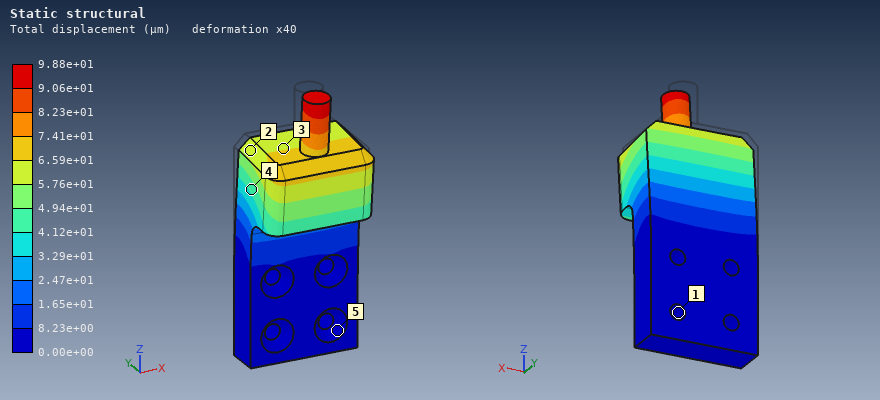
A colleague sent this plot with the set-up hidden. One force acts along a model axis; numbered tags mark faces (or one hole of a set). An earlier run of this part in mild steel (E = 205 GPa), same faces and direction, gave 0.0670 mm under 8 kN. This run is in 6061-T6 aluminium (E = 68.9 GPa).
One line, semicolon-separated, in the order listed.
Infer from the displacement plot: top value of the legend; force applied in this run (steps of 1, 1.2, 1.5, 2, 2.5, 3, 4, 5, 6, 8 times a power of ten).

9.88e+01 µm; 4 kN
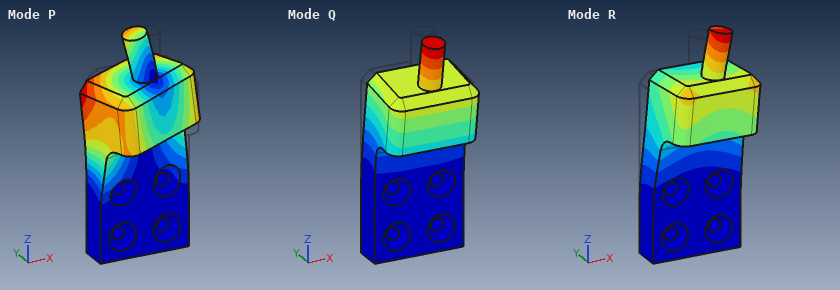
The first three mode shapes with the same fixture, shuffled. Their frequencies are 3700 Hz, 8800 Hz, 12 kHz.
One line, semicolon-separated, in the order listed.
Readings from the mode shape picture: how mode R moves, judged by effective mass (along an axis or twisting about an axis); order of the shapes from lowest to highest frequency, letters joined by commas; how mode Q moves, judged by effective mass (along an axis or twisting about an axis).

along X; Q, R, P; along Y
